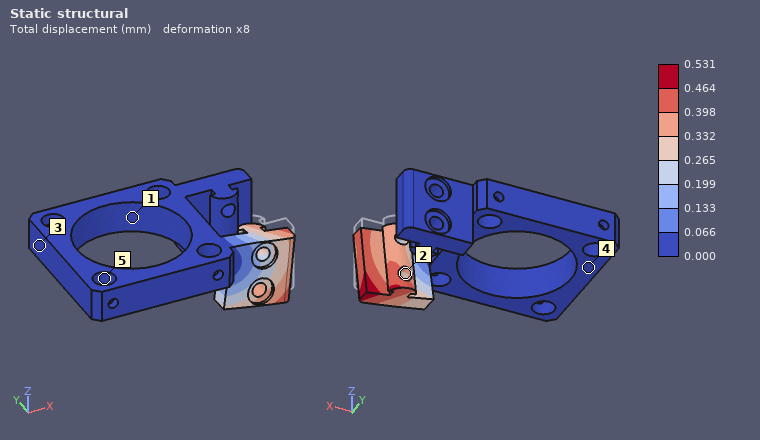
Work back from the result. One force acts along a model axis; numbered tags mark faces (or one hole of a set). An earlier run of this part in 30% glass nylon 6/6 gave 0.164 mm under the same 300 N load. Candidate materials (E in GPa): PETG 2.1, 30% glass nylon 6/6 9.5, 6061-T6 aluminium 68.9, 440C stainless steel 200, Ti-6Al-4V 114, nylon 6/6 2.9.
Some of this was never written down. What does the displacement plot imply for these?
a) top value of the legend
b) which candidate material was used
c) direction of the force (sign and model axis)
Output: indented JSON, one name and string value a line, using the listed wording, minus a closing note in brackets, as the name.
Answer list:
{
  "top value of the legend": "0.531 mm",
  "which candidate material was used": "nylon 6/6",
  "direction of the force": "-Z"
}
